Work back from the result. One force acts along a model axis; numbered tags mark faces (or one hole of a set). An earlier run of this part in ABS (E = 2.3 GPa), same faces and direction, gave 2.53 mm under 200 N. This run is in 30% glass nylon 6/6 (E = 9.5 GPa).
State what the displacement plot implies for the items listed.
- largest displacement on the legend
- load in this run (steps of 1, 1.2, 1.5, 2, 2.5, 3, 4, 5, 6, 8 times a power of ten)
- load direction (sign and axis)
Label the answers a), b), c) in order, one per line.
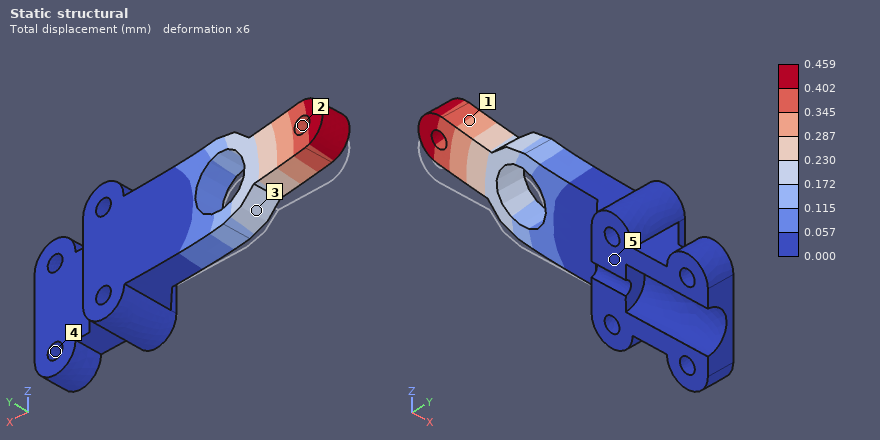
a) 0.459 mm
b) 150 N
c) +Z
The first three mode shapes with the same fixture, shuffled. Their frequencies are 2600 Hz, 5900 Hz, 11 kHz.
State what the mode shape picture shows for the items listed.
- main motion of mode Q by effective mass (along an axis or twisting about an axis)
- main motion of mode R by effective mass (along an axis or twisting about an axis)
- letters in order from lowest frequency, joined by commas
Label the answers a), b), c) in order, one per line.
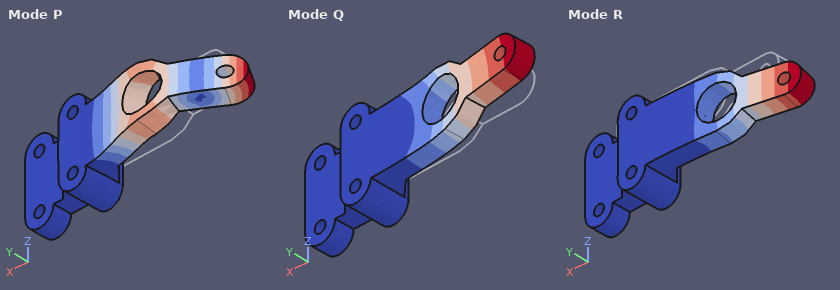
a) along Z
b) along Y
c) R, Q, P
